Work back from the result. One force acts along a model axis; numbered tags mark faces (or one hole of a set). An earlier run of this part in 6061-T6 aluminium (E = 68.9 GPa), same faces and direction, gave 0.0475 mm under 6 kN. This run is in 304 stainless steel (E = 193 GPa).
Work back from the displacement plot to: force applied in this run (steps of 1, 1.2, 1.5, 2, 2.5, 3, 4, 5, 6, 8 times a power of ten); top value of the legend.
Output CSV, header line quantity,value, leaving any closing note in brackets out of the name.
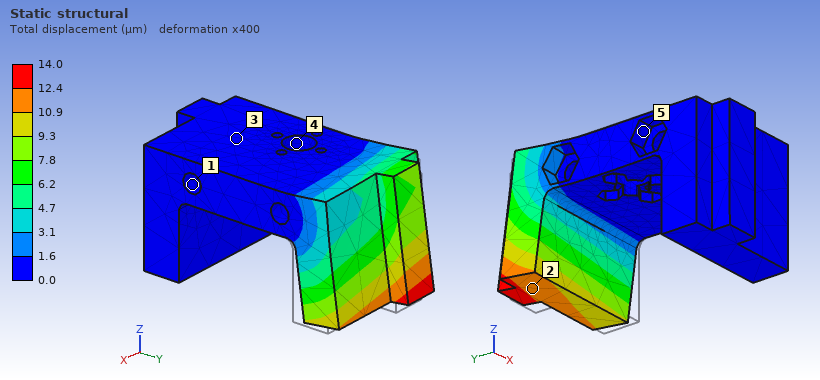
quantity,value
force applied in this run,5 kN
top value of the legend,14.0 µm
